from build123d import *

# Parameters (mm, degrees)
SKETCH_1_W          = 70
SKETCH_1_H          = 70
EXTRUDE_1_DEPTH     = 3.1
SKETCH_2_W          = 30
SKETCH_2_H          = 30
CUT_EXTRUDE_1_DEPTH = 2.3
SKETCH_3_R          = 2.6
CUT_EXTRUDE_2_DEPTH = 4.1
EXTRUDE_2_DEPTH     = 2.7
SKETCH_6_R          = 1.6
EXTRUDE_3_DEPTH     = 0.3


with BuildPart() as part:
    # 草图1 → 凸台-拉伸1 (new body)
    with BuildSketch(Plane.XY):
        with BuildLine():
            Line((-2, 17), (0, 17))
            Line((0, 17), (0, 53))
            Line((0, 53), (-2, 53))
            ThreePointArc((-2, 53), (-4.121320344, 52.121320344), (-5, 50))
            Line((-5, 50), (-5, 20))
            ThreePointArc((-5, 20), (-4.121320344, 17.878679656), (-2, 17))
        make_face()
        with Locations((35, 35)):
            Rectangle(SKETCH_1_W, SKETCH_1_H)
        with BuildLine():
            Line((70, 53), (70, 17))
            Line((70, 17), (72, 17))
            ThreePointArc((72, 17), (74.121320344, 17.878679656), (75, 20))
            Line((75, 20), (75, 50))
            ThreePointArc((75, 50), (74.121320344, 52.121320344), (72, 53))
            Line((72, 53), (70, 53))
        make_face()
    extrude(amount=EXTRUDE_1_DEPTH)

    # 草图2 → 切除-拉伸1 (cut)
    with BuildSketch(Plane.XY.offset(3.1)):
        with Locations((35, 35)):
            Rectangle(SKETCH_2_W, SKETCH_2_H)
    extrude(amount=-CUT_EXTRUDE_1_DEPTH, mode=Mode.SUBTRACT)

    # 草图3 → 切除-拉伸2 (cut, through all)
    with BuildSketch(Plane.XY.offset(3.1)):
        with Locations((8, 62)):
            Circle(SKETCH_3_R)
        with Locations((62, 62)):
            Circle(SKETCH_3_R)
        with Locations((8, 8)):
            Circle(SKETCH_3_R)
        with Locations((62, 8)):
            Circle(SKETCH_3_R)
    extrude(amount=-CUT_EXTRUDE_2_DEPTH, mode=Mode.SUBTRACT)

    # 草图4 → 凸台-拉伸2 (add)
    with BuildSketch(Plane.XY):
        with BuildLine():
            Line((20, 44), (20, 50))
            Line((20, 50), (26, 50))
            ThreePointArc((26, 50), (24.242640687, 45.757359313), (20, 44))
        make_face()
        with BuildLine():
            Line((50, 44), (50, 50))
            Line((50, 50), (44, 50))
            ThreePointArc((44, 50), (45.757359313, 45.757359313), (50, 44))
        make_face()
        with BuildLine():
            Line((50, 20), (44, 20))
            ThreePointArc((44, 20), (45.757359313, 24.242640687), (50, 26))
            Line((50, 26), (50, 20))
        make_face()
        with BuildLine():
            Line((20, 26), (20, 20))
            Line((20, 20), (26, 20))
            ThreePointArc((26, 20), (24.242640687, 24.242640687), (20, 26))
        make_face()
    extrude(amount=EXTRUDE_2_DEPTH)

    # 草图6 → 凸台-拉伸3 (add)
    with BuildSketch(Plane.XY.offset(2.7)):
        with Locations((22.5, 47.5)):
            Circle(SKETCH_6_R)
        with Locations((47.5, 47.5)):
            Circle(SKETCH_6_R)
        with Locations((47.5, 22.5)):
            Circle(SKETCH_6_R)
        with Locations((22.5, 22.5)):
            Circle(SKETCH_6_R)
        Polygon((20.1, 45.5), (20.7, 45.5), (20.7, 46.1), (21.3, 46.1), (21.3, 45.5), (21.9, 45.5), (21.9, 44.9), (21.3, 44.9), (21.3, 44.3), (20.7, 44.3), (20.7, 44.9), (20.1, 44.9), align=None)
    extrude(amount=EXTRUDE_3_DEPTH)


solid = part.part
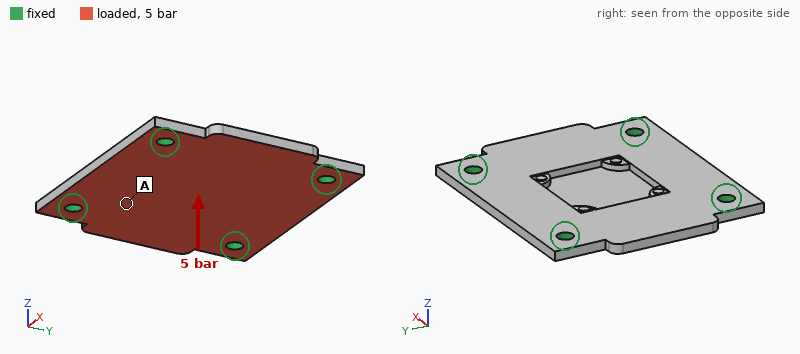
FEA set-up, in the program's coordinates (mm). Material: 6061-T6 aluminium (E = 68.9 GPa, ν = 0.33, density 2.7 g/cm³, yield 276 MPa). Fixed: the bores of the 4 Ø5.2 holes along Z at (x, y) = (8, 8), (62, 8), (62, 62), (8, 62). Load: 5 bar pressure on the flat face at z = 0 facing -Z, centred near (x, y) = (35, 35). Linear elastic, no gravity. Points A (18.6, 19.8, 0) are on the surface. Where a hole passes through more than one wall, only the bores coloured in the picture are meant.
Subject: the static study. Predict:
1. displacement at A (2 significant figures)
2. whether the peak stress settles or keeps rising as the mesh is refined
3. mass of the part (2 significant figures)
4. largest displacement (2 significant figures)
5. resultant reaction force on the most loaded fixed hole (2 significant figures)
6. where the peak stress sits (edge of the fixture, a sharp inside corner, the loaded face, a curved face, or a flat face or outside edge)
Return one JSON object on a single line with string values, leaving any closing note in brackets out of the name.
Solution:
{"displacement at A": "0.083 mm", "whether the peak stress settles or keeps rising as the mesh is refined": "keeps rising", "mass of the part": "38 g", "largest displacement": "0.32 mm", "resultant reaction force on the most loaded fixed hole": "710 N", "where the peak stress sits": "edge of the fixture"}
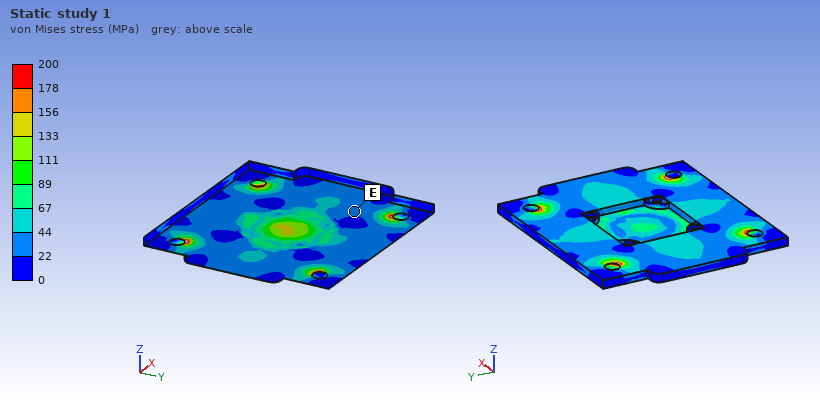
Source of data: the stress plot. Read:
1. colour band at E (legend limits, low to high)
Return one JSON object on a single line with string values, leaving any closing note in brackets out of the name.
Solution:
{"colour band at E": "22 to 44 MPa"}
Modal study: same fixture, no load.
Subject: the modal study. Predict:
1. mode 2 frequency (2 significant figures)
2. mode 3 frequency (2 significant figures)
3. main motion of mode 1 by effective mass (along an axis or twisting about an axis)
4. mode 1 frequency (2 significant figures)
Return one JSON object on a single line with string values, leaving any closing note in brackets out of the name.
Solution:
{"mode 2 frequency": "5500 Hz", "mode 3 frequency": "5600 Hz", "main motion of mode 1 by effective mass": "along Z", "mode 1 frequency": "4600 Hz"}
